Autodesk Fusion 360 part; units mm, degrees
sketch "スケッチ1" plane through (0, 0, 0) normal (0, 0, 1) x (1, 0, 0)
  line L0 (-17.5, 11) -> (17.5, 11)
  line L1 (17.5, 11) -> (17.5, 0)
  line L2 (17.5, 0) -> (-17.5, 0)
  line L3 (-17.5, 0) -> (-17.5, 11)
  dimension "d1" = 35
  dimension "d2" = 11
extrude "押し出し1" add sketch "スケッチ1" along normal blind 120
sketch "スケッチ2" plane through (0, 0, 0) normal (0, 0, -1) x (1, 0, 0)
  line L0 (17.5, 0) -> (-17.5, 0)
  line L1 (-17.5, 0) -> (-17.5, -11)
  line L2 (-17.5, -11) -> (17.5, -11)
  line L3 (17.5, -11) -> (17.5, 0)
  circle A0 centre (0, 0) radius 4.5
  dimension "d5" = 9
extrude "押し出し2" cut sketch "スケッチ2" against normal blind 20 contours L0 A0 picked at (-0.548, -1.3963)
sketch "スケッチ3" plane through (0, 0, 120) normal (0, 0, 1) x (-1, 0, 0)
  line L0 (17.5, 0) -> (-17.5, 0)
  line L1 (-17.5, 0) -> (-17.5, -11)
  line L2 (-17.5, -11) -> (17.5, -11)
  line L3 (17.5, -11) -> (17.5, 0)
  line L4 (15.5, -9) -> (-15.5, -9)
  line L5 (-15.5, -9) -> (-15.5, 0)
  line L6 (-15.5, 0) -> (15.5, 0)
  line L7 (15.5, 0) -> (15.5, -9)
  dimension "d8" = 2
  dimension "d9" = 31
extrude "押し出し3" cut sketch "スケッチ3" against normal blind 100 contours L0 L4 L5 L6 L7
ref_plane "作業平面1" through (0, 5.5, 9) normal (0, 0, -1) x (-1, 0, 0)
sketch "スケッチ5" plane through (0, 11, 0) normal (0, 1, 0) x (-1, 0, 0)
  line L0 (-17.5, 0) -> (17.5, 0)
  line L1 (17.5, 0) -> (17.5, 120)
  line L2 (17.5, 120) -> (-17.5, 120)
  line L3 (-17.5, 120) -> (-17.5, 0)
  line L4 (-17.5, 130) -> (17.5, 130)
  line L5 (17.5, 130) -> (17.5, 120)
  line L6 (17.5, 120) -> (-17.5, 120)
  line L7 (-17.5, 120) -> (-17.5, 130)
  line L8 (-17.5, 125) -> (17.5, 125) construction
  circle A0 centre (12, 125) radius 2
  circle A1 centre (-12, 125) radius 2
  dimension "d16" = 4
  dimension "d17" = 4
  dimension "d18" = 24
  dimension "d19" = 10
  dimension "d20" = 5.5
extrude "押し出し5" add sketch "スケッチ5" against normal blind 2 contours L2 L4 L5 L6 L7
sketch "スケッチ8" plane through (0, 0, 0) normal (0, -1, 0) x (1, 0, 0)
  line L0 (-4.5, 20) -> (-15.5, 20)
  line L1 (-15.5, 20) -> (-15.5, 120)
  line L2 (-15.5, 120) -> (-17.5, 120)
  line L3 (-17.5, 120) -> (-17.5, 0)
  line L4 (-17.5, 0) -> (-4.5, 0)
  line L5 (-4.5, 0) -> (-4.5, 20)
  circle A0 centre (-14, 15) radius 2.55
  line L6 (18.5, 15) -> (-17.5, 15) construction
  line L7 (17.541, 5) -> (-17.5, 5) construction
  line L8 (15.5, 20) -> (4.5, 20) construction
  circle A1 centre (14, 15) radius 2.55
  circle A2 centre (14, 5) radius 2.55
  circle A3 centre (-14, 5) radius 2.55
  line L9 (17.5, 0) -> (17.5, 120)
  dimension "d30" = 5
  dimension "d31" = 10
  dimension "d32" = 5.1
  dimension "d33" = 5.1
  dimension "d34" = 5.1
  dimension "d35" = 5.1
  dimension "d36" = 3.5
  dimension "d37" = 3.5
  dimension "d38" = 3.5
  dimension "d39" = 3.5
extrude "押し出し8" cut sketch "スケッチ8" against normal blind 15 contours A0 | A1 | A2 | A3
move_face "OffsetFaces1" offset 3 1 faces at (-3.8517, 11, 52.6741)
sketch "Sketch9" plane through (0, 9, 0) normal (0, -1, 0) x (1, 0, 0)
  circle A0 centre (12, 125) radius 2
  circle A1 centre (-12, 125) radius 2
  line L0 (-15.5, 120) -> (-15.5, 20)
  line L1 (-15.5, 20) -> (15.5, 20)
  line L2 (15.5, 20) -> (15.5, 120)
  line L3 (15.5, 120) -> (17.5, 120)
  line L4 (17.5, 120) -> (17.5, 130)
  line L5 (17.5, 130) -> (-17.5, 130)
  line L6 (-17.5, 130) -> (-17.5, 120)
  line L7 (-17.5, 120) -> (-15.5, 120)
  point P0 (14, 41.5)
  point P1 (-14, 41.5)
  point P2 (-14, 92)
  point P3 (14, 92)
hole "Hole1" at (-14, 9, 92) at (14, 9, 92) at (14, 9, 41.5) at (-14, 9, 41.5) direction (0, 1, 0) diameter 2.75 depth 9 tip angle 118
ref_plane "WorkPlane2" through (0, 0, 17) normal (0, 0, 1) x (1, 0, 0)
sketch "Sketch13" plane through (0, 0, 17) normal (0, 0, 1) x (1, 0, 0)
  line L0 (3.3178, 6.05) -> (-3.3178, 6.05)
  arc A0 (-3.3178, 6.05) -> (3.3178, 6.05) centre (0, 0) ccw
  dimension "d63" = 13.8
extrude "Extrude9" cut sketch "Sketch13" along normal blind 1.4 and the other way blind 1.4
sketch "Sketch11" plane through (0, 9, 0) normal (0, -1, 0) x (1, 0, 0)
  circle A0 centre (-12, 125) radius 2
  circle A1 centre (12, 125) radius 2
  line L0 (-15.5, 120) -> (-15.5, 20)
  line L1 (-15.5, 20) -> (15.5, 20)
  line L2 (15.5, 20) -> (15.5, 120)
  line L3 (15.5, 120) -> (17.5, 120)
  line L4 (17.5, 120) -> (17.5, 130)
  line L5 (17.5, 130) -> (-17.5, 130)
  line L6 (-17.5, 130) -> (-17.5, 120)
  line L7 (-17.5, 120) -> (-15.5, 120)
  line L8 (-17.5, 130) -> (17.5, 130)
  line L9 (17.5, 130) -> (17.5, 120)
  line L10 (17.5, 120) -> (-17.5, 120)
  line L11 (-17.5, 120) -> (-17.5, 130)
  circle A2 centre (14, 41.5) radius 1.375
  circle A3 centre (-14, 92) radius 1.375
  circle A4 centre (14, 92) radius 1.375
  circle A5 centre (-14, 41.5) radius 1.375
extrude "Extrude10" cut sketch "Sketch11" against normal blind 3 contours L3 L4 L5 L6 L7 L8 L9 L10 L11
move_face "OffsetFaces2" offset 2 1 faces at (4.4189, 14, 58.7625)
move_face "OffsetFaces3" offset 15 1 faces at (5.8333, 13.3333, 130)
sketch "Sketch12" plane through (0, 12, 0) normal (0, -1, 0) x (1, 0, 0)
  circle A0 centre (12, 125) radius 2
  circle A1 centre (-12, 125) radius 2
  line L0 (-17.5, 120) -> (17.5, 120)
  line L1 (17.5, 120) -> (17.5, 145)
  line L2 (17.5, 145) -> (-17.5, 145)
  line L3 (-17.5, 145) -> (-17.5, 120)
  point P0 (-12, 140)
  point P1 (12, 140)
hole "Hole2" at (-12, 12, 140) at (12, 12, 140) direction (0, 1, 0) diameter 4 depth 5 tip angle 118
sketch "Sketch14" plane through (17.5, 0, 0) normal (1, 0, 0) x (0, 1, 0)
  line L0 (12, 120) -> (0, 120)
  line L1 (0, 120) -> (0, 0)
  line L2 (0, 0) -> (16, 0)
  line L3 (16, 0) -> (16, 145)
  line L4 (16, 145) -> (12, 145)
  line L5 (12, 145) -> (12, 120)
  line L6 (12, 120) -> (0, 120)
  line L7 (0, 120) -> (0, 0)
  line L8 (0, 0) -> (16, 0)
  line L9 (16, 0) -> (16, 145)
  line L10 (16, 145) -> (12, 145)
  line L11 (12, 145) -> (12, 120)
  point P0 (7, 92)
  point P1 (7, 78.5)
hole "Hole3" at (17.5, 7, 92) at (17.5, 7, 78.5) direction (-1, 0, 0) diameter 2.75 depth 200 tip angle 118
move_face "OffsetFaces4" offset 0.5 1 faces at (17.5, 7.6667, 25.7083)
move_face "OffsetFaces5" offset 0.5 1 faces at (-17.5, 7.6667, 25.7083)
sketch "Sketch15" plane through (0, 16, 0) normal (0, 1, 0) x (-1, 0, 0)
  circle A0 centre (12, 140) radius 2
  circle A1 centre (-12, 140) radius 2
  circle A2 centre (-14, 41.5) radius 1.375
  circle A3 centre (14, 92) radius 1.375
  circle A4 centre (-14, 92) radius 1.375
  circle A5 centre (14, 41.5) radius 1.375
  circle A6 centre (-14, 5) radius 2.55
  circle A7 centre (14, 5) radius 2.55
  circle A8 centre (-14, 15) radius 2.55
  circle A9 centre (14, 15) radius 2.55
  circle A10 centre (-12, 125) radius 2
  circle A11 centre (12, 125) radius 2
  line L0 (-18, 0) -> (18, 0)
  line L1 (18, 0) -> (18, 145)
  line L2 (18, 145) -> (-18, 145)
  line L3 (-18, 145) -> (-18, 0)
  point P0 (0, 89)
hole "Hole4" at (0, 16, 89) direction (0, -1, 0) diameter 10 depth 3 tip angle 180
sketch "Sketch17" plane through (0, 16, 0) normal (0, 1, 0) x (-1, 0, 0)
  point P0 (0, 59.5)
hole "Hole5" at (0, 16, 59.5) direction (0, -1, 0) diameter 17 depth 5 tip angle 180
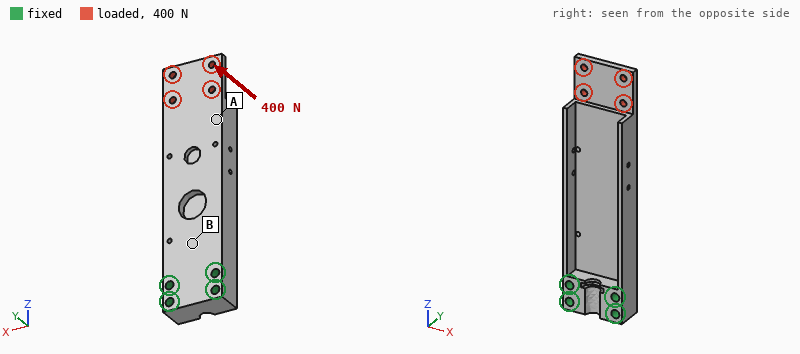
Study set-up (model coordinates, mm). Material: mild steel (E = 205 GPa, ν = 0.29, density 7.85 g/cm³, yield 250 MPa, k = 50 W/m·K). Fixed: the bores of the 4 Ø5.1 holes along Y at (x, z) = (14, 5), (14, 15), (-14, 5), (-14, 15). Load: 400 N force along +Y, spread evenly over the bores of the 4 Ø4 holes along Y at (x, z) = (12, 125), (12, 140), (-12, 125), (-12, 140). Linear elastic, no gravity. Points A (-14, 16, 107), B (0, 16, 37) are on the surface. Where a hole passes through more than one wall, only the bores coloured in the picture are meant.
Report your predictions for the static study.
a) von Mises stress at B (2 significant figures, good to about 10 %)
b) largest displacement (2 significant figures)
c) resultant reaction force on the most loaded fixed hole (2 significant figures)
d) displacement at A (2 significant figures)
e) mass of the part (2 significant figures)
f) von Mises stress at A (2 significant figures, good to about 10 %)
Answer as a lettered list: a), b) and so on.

a) 42 MPa
b) 0.38 mm
c) 490 N
d) 0.20 mm
e) 320 g
f) 16 MPa
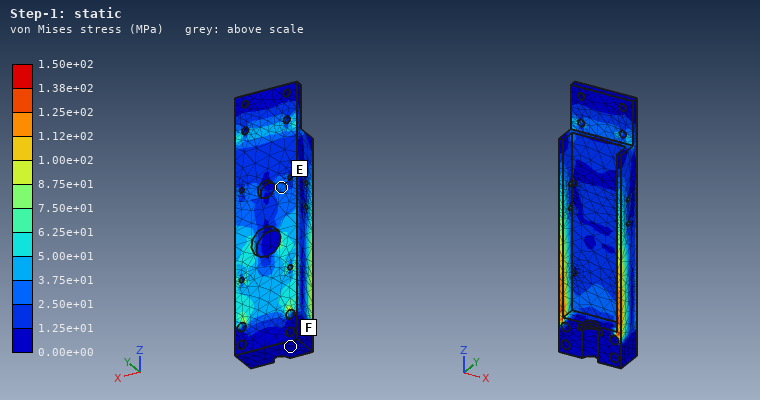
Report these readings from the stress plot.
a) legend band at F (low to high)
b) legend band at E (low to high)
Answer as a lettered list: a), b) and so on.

a) 0.00e+00 to 1.25e+01 MPa
b) 2.50e+01 to 3.75e+01 MPa
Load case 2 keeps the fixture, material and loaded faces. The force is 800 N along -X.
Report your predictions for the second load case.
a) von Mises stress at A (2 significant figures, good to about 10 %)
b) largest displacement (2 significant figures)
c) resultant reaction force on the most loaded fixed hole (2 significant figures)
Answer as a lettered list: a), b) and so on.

a) 11 MPa
b) 73 µm
c) 3.0 kN
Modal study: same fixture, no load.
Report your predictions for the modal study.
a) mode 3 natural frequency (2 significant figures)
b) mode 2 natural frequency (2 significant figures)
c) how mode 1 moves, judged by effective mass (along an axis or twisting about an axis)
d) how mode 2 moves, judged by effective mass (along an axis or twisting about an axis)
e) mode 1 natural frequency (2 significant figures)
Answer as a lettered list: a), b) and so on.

a) 2500 Hz
b) 2100 Hz
c) along Y
d) along X
e) 710 Hz
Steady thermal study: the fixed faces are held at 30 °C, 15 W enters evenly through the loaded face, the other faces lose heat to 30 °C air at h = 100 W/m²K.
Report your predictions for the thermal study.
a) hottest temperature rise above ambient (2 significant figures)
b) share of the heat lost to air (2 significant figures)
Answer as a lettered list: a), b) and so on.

a) 40 K
b) 95 %
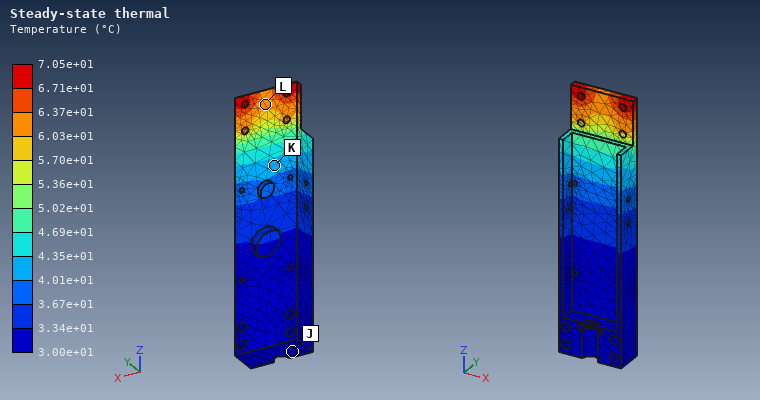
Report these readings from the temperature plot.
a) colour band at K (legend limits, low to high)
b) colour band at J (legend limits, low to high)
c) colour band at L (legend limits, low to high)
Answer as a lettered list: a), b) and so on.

a) 4.01e+01 to 4.35e+01 °C
b) 3.00e+01 to 3.34e+01 °C
c) 6.03e+01 to 6.37e+01 °C
